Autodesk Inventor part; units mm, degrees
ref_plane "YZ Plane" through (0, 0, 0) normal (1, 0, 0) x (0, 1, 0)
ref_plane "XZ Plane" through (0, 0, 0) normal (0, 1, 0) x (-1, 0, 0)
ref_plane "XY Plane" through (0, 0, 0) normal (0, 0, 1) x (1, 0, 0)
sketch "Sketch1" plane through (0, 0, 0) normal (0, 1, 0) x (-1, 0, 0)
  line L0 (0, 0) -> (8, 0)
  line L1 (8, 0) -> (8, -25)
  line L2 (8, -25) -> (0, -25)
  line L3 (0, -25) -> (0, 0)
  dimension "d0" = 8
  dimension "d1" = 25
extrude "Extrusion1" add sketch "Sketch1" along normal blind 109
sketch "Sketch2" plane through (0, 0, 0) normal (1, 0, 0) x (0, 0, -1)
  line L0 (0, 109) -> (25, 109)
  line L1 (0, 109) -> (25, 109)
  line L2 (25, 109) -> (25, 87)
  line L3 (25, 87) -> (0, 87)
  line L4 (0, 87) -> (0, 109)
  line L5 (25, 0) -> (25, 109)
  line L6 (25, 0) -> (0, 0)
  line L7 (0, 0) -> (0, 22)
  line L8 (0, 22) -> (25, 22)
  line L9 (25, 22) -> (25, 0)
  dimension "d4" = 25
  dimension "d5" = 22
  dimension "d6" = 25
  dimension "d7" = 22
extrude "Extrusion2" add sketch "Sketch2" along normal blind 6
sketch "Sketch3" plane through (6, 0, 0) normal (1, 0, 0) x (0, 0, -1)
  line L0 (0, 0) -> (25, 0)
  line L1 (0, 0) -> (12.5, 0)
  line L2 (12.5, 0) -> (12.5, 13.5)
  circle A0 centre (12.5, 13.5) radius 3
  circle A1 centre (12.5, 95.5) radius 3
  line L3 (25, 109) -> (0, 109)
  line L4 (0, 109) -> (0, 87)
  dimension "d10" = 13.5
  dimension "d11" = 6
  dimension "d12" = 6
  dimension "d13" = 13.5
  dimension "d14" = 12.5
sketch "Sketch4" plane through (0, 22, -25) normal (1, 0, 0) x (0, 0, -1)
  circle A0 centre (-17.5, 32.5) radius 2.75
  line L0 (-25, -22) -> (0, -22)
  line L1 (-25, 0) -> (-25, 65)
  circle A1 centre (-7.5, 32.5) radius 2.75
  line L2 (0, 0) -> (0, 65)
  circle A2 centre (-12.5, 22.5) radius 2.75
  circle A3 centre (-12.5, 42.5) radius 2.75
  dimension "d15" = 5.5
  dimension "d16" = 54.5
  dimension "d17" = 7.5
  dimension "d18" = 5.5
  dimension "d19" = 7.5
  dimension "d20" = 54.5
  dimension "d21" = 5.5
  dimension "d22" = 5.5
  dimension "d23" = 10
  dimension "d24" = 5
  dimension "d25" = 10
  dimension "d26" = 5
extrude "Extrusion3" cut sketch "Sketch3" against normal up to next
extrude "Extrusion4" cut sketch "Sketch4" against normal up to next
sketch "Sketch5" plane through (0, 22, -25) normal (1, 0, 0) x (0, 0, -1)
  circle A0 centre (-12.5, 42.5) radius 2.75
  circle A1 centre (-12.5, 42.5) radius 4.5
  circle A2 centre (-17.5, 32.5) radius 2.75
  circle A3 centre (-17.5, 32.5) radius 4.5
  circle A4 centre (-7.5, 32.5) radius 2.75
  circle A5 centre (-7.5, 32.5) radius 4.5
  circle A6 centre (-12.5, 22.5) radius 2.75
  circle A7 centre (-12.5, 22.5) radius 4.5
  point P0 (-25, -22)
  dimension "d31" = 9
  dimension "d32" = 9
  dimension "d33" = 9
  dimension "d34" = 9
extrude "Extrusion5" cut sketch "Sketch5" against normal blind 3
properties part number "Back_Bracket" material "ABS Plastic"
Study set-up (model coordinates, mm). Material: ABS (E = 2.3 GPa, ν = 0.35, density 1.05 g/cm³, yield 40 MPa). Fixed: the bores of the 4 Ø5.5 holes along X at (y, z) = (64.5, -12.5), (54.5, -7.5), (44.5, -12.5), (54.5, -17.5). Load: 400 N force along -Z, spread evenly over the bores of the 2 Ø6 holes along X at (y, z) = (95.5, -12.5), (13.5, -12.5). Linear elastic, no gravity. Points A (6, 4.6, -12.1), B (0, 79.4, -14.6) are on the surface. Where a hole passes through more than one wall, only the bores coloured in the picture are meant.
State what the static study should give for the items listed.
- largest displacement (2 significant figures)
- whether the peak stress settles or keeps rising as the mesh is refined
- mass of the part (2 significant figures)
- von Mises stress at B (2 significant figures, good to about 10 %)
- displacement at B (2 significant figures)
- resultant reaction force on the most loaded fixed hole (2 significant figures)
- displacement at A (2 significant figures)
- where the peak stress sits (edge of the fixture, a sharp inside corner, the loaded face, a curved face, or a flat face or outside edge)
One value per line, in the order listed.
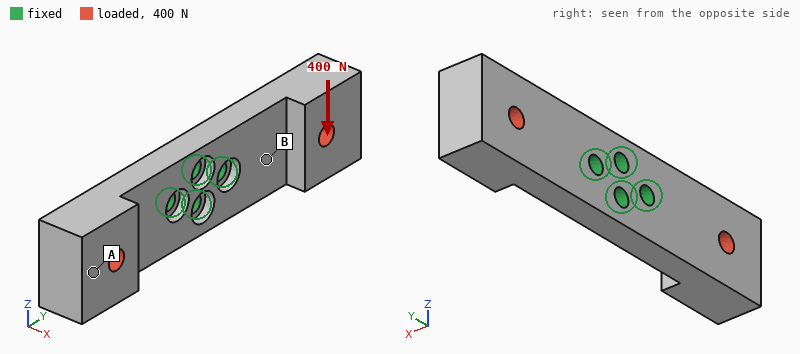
0.34 mm
keeps rising
28 g
4.5 MPa
0.095 mm
290 N
0.30 mm
edge of the fixture
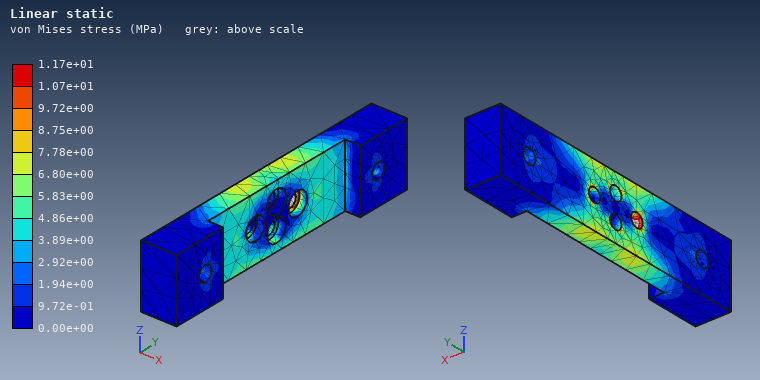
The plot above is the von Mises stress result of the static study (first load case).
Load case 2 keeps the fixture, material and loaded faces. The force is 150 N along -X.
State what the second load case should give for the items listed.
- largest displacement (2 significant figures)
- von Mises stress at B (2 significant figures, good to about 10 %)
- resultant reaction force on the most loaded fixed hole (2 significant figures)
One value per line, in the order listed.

0.68 mm
3.9 MPa
210 N
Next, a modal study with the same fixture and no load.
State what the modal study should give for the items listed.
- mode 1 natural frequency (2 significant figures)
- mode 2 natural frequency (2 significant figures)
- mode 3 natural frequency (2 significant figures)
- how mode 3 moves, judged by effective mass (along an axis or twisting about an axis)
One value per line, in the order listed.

650 Hz
650 Hz
1400 Hz
twisting about X
